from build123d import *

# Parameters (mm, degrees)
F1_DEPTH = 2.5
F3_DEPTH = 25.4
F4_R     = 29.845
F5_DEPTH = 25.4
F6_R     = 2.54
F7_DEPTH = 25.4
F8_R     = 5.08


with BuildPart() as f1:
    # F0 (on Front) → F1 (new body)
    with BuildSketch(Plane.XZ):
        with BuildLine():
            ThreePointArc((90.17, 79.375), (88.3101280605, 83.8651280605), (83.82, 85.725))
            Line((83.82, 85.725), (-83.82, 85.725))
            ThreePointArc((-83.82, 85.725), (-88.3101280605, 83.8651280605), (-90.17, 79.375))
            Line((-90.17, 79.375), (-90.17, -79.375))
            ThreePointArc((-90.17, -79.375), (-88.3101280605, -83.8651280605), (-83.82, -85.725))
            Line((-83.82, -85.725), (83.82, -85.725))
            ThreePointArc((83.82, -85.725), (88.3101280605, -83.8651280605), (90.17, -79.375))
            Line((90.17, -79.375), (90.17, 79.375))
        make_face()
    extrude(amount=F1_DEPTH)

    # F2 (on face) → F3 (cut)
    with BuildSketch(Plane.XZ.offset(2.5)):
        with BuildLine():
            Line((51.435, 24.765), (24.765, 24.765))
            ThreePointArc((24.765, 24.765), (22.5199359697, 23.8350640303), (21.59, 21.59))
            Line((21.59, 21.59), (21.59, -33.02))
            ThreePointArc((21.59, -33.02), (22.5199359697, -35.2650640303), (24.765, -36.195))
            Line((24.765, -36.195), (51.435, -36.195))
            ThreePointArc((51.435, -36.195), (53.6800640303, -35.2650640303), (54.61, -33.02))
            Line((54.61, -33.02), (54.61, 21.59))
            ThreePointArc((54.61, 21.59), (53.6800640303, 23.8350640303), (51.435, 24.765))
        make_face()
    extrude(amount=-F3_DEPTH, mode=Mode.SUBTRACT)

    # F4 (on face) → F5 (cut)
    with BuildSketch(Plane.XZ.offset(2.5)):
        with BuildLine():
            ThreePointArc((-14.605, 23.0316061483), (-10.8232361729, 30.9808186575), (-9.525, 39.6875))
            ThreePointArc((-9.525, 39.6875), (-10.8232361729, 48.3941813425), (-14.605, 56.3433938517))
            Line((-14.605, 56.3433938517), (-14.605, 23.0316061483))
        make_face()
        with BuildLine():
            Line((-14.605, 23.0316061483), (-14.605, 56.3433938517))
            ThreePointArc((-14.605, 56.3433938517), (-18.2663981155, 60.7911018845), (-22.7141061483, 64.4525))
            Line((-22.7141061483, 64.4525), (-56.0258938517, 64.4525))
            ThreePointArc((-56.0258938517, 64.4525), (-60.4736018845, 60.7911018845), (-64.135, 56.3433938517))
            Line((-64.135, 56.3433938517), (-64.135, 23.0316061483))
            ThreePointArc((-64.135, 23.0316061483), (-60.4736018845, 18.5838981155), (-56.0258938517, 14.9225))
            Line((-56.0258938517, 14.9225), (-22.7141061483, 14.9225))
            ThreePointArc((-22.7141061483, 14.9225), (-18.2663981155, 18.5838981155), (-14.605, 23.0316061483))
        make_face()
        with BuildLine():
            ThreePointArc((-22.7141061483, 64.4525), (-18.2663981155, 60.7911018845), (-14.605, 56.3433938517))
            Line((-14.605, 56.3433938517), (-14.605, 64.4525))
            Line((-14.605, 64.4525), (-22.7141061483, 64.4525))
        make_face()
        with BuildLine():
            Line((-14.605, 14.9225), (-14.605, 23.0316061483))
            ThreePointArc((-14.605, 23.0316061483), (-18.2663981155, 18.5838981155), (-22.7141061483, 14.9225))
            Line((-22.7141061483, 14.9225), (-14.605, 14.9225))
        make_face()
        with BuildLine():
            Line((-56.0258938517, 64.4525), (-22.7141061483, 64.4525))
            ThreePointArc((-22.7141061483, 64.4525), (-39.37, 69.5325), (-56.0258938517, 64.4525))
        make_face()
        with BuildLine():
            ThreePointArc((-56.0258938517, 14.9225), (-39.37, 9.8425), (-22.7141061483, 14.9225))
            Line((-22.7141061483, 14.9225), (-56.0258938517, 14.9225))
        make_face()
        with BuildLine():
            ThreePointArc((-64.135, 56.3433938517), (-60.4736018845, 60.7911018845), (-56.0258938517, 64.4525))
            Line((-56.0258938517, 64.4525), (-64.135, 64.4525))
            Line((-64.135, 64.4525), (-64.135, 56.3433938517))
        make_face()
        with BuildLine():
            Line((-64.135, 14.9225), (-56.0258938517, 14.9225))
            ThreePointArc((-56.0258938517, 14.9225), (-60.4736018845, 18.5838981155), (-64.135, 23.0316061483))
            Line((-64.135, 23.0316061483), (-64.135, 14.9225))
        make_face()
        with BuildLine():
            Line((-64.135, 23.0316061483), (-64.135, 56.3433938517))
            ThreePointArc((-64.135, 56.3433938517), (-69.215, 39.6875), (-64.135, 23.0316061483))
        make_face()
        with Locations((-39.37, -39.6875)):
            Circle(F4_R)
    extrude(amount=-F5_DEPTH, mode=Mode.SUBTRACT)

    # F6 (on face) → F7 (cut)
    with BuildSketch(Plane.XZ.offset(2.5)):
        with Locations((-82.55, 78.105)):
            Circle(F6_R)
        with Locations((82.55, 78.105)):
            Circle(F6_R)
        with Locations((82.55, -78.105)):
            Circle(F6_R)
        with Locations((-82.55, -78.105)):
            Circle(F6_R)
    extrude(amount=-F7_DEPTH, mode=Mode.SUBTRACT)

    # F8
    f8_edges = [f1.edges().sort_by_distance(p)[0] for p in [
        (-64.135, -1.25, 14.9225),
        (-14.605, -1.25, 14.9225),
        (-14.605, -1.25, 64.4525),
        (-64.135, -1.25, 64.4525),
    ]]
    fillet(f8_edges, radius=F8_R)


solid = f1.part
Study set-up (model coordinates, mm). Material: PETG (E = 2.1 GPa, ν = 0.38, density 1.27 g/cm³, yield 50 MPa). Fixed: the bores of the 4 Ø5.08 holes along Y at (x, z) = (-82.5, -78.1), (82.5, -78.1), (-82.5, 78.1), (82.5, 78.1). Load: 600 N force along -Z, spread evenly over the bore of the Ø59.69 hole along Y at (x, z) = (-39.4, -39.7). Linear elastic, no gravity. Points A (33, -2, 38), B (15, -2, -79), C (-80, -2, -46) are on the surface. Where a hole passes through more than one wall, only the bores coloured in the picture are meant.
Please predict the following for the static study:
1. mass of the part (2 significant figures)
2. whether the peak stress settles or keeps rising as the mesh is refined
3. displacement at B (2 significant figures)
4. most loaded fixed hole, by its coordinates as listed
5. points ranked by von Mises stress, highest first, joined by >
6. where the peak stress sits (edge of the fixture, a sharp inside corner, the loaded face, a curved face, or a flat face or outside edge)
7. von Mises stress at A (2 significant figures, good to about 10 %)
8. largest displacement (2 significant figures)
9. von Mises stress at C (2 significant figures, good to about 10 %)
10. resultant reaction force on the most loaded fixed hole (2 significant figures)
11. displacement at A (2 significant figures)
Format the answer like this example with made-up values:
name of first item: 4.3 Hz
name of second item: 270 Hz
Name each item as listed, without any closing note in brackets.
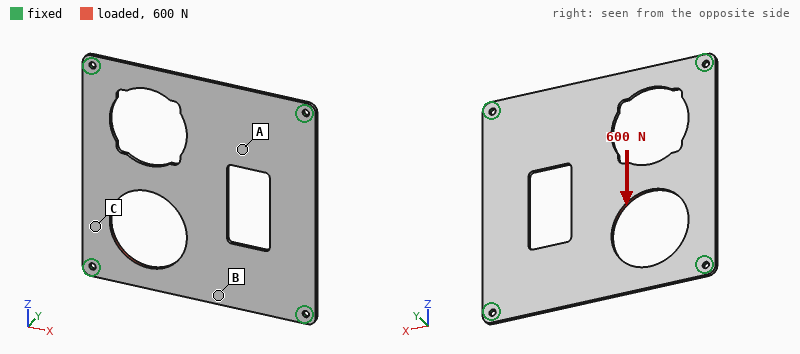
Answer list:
mass of the part: 73 g
whether the peak stress settles or keeps rising as the mesh is refined: keeps rising
displacement at B: 0.21 mm
most loaded fixed hole, by its coordinates as listed: (-82.5, -78.1)
points ranked by von Mises stress, highest first, joined by >: C > A > B
where the peak stress sits: edge of the fixture
von Mises stress at A: 2.2 MPa
largest displacement: 0.33 mm
von Mises stress at C: 3.7 MPa
resultant reaction force on the most loaded fixed hole: 240 N
displacement at A: 0.12 mm
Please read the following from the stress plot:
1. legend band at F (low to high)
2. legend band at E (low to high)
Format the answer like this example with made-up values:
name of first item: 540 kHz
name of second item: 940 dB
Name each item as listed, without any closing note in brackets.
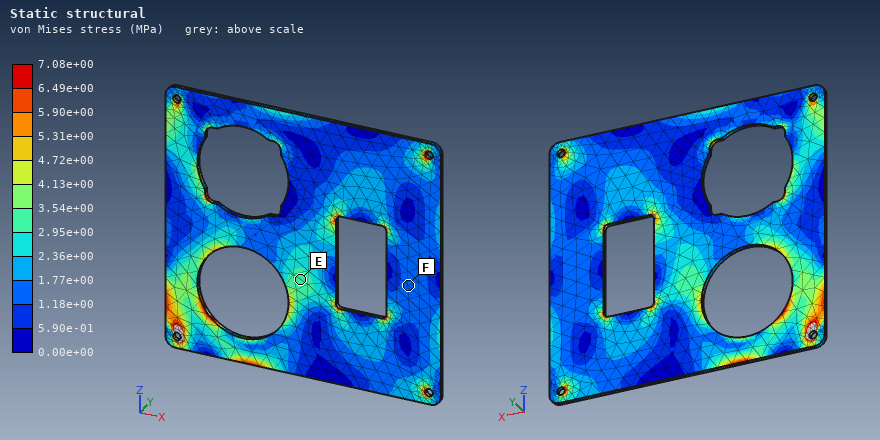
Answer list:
legend band at F: 1.18e+00 to 1.77e+00 MPa
legend band at E: 2.95e+00 to 3.54e+00 MPa
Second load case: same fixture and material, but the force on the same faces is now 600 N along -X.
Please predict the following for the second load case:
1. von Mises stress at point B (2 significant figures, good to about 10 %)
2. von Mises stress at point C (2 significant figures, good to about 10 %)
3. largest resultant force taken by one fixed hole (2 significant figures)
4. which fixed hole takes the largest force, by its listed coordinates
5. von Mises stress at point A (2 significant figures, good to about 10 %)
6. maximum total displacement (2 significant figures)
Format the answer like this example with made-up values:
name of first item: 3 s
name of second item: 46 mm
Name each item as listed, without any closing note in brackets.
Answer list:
von Mises stress at point B: 0.94 MPa
von Mises stress at point C: 2.2 MPa
largest resultant force taken by one fixed hole: 240 N
which fixed hole takes the largest force, by its listed coordinates: (-82.5, -78.1)
von Mises stress at point A: 1.9 MPa
maximum total displacement: 0.25 mm
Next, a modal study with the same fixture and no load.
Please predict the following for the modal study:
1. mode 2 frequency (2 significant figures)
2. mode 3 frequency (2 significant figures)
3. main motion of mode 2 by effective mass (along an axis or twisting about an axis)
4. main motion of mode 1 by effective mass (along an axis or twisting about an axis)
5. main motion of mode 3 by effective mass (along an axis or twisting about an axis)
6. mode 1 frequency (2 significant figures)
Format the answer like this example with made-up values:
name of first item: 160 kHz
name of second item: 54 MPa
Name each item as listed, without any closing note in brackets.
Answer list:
mode 2 frequency: 130 Hz
mode 3 frequency: 140 Hz
main motion of mode 2 by effective mass: twisting about X
main motion of mode 1 by effective mass: along Y
main motion of mode 3 by effective mass: twisting about Z
mode 1 frequency: 78 Hz
